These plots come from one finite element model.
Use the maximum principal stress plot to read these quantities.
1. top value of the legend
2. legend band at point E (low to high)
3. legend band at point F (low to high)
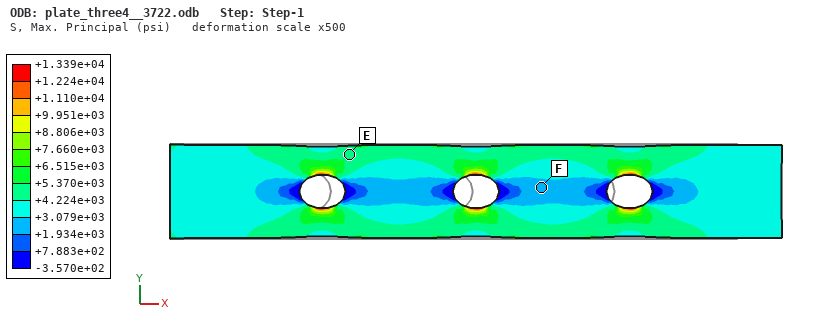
+1.339e+04 psi
+4.224e+03 to +5.370e+03 psi
+1.934e+03 to +3.079e+03 psi
